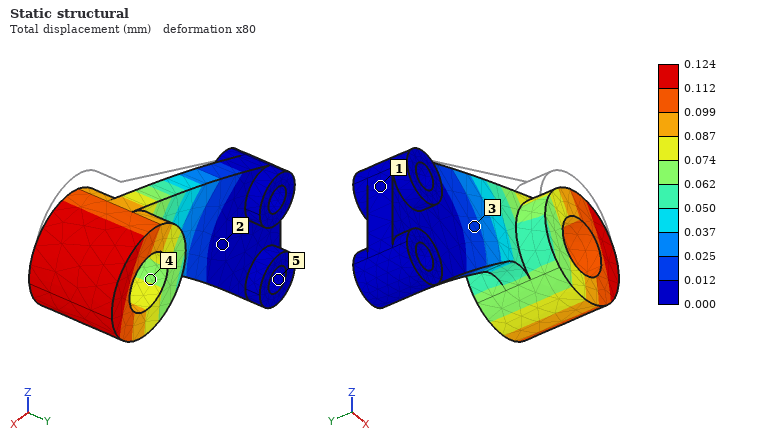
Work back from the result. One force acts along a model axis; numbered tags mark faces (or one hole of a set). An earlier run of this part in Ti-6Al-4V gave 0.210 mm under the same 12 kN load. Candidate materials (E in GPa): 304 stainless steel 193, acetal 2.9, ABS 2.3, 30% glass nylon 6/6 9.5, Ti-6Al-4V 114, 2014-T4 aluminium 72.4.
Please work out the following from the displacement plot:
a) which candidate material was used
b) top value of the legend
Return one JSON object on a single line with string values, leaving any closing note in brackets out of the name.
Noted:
{"which candidate material was used": "304 stainless steel", "top value of the legend": "0.124 mm"}
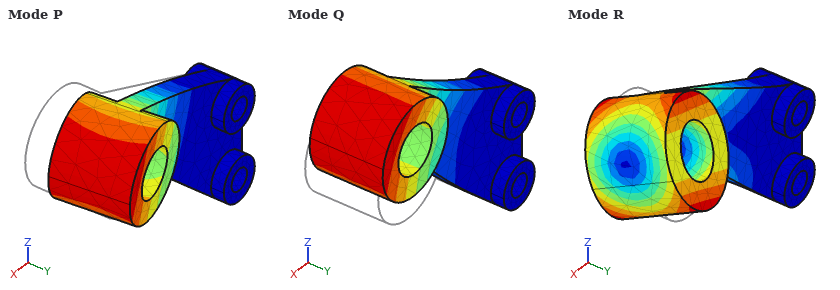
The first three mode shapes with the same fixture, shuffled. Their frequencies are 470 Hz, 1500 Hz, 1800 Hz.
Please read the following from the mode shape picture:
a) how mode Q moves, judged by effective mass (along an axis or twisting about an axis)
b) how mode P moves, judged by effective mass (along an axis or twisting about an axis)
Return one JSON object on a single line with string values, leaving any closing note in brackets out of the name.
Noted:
{"how mode Q moves, judged by effective mass": "along Z", "how mode P moves, judged by effective mass": "along Y"}
